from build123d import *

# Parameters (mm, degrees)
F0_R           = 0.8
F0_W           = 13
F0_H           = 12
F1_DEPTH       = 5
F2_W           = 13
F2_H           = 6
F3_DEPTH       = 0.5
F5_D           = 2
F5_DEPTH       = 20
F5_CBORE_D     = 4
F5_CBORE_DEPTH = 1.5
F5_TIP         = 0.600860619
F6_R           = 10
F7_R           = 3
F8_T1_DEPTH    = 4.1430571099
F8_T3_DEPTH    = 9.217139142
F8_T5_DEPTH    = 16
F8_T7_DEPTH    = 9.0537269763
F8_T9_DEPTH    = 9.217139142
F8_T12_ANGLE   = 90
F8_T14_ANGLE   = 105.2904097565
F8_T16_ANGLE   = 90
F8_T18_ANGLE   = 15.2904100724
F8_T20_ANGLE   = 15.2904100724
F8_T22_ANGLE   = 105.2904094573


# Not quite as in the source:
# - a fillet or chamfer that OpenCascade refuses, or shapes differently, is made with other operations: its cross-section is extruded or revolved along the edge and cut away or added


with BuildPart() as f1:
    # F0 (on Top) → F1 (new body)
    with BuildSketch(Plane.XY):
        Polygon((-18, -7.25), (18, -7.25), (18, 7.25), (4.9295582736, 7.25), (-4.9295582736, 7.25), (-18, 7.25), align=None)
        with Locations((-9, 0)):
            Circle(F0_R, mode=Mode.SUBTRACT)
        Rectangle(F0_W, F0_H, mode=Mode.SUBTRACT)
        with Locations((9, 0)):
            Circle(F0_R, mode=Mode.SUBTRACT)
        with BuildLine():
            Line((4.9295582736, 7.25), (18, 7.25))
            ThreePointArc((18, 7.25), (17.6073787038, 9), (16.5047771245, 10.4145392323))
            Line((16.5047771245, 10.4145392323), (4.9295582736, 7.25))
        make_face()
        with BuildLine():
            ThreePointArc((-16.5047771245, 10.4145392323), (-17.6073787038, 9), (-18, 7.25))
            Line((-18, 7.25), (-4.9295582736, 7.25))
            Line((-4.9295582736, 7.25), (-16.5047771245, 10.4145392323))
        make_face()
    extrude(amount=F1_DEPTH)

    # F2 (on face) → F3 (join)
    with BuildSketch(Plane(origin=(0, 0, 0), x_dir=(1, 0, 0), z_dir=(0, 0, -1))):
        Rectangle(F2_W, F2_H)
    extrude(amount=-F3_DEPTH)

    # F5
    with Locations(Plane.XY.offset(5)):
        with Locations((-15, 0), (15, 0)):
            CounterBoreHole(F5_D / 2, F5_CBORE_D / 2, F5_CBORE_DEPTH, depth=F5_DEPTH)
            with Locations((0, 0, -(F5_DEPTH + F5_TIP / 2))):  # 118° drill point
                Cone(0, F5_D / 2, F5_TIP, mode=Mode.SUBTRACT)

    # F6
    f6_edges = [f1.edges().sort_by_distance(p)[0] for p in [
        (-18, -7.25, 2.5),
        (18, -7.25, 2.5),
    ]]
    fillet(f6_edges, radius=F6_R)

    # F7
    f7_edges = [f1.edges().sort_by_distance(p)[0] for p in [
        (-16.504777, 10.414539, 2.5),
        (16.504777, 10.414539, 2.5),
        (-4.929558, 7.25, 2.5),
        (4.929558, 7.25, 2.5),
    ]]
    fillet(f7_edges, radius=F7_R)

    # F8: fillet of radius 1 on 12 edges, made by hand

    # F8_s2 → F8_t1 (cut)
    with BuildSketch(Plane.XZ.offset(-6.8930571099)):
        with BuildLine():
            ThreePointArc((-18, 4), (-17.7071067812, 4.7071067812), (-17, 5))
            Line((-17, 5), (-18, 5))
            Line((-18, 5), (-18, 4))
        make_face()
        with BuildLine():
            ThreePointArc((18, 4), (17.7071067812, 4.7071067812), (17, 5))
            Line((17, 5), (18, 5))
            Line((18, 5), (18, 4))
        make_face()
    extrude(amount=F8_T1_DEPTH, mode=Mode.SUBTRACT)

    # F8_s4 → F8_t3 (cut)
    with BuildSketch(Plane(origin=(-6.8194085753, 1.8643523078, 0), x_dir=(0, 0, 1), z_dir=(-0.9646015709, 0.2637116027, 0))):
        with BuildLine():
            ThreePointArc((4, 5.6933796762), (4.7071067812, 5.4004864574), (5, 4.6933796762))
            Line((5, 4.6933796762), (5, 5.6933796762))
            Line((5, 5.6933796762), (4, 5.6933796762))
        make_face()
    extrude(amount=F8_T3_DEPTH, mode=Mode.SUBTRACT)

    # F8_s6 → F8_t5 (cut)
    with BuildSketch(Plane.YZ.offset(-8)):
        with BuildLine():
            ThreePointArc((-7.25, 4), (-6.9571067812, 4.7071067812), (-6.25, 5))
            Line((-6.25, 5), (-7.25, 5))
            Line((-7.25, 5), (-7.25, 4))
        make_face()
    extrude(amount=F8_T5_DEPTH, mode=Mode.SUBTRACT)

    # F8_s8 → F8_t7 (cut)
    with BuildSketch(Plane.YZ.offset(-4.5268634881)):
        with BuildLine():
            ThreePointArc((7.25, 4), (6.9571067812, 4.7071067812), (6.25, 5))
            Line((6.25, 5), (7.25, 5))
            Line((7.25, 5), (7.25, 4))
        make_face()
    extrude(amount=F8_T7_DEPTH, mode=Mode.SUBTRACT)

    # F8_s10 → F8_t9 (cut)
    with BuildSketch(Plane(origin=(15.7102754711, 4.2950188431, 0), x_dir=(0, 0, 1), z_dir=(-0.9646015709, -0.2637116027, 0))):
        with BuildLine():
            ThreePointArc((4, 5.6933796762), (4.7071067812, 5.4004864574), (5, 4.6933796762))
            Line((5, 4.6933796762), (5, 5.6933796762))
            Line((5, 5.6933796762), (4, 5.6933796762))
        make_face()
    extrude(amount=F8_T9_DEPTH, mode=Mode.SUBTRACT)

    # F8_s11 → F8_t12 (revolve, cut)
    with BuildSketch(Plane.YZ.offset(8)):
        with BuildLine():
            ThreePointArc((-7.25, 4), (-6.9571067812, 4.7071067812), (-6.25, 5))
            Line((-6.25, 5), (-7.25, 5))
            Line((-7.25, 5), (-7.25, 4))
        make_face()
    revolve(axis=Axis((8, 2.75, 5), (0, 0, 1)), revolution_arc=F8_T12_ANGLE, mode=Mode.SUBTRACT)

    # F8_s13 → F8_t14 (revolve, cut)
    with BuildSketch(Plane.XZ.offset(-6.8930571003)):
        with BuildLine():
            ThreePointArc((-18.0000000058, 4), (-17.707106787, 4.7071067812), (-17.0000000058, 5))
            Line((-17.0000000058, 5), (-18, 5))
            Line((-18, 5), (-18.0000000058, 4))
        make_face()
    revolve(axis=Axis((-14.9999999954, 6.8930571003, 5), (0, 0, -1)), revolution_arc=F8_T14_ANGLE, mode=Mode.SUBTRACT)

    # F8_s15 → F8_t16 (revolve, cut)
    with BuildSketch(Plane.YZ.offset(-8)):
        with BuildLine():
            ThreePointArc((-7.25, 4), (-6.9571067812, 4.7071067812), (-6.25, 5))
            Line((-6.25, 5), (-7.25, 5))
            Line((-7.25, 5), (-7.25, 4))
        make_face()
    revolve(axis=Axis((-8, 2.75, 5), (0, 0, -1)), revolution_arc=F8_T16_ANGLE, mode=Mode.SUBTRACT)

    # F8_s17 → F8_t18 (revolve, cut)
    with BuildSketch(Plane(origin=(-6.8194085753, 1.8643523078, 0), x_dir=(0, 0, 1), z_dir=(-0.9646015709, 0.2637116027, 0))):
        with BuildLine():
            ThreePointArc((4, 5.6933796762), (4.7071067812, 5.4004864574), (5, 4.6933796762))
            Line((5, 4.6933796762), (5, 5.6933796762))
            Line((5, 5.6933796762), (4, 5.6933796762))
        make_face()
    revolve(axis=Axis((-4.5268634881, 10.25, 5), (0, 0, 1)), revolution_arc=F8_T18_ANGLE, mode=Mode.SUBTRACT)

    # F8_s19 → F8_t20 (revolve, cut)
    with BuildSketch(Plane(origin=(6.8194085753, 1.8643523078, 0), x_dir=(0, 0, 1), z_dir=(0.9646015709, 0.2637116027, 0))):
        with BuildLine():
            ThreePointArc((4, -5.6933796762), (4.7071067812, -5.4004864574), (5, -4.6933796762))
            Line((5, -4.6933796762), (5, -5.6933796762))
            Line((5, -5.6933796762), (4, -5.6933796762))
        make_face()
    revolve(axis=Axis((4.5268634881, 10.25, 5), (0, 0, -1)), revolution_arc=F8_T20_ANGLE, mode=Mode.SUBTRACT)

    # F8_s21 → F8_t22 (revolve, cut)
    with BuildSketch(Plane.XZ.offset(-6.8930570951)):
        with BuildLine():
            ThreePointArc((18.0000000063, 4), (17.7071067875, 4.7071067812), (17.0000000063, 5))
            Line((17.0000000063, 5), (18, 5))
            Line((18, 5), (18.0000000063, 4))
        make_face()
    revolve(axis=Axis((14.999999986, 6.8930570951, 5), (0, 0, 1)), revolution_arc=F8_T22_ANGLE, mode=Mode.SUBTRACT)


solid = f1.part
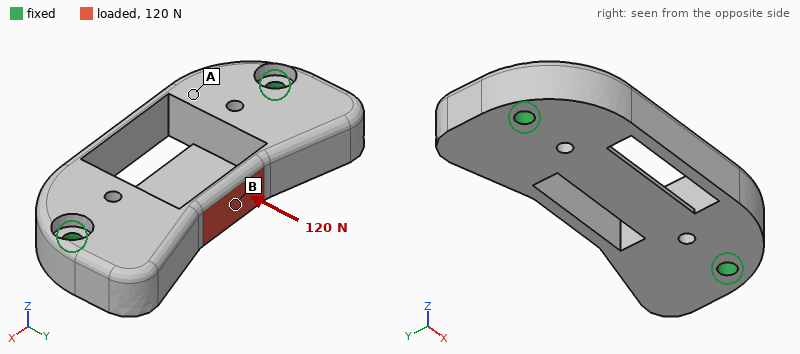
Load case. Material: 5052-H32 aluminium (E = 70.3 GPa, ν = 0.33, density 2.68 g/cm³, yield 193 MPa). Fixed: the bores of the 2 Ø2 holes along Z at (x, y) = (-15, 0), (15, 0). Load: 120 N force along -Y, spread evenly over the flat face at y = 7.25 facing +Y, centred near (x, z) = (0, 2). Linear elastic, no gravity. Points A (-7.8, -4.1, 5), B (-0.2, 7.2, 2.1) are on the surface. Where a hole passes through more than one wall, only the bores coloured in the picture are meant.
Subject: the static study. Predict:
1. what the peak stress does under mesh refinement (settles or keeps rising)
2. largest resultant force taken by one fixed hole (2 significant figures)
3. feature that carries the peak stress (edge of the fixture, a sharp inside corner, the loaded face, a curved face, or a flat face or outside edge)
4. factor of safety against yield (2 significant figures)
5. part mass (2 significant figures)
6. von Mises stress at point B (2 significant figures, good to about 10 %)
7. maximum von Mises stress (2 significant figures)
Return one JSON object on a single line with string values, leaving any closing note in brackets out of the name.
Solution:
{"what the peak stress does under mesh refinement": "settles", "largest resultant force taken by one fixed hole": "61 N", "feature that carries the peak stress": "the loaded face", "factor of safety against yield": "2.3", "part mass": "4.7 g", "von Mises stress at point B": "75 MPa", "maximum von Mises stress": "83 MPa"}
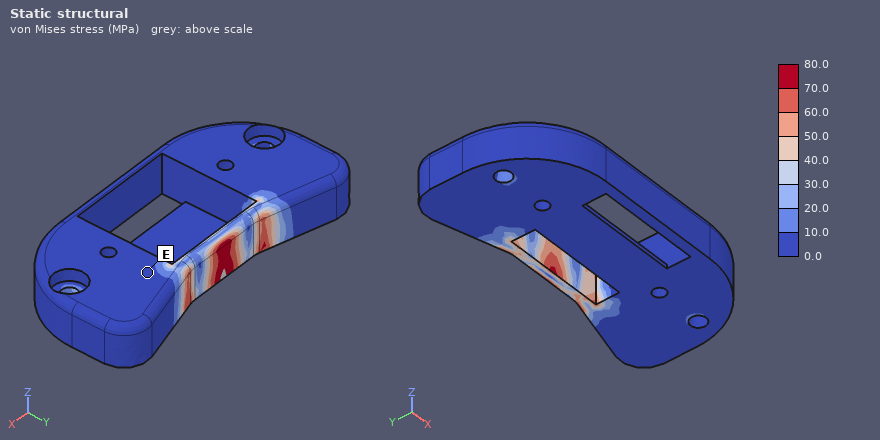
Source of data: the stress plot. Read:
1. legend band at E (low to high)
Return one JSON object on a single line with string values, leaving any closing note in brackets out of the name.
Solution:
{"legend band at E": "0.0 to 10.0 MPa"}
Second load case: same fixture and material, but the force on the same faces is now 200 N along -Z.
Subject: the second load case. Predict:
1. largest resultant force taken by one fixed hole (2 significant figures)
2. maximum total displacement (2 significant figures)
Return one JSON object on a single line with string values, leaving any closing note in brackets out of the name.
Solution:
{"largest resultant force taken by one fixed hole": "100 N", "maximum total displacement": "29 µm"}
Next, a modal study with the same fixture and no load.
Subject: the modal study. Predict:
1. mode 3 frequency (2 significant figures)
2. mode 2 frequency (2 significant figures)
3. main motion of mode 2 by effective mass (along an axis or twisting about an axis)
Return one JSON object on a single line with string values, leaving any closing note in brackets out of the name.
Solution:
{"mode 3 frequency": "21 kHz", "mode 2 frequency": "20 kHz", "main motion of mode 2 by effective mass": "along Z"}
